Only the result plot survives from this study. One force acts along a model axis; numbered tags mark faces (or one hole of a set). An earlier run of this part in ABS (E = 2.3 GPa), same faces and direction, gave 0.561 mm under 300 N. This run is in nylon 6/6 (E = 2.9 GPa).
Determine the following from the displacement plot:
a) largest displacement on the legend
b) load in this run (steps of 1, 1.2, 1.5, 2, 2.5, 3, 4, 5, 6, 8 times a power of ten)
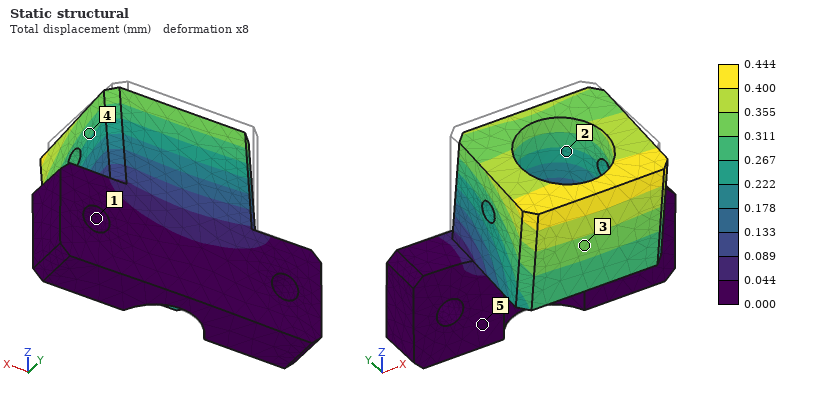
0.444 mm
300 N
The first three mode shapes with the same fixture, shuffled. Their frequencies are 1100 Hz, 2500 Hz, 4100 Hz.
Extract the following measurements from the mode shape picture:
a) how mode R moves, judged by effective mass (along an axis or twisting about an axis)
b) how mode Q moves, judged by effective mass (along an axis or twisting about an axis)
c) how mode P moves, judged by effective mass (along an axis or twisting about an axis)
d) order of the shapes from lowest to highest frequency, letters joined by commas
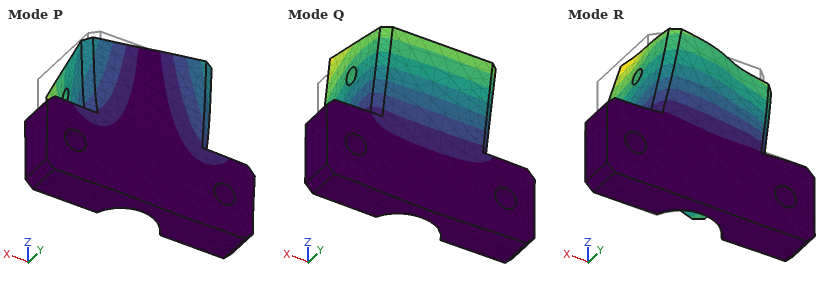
along X
along Y
along X
Q, P, R
